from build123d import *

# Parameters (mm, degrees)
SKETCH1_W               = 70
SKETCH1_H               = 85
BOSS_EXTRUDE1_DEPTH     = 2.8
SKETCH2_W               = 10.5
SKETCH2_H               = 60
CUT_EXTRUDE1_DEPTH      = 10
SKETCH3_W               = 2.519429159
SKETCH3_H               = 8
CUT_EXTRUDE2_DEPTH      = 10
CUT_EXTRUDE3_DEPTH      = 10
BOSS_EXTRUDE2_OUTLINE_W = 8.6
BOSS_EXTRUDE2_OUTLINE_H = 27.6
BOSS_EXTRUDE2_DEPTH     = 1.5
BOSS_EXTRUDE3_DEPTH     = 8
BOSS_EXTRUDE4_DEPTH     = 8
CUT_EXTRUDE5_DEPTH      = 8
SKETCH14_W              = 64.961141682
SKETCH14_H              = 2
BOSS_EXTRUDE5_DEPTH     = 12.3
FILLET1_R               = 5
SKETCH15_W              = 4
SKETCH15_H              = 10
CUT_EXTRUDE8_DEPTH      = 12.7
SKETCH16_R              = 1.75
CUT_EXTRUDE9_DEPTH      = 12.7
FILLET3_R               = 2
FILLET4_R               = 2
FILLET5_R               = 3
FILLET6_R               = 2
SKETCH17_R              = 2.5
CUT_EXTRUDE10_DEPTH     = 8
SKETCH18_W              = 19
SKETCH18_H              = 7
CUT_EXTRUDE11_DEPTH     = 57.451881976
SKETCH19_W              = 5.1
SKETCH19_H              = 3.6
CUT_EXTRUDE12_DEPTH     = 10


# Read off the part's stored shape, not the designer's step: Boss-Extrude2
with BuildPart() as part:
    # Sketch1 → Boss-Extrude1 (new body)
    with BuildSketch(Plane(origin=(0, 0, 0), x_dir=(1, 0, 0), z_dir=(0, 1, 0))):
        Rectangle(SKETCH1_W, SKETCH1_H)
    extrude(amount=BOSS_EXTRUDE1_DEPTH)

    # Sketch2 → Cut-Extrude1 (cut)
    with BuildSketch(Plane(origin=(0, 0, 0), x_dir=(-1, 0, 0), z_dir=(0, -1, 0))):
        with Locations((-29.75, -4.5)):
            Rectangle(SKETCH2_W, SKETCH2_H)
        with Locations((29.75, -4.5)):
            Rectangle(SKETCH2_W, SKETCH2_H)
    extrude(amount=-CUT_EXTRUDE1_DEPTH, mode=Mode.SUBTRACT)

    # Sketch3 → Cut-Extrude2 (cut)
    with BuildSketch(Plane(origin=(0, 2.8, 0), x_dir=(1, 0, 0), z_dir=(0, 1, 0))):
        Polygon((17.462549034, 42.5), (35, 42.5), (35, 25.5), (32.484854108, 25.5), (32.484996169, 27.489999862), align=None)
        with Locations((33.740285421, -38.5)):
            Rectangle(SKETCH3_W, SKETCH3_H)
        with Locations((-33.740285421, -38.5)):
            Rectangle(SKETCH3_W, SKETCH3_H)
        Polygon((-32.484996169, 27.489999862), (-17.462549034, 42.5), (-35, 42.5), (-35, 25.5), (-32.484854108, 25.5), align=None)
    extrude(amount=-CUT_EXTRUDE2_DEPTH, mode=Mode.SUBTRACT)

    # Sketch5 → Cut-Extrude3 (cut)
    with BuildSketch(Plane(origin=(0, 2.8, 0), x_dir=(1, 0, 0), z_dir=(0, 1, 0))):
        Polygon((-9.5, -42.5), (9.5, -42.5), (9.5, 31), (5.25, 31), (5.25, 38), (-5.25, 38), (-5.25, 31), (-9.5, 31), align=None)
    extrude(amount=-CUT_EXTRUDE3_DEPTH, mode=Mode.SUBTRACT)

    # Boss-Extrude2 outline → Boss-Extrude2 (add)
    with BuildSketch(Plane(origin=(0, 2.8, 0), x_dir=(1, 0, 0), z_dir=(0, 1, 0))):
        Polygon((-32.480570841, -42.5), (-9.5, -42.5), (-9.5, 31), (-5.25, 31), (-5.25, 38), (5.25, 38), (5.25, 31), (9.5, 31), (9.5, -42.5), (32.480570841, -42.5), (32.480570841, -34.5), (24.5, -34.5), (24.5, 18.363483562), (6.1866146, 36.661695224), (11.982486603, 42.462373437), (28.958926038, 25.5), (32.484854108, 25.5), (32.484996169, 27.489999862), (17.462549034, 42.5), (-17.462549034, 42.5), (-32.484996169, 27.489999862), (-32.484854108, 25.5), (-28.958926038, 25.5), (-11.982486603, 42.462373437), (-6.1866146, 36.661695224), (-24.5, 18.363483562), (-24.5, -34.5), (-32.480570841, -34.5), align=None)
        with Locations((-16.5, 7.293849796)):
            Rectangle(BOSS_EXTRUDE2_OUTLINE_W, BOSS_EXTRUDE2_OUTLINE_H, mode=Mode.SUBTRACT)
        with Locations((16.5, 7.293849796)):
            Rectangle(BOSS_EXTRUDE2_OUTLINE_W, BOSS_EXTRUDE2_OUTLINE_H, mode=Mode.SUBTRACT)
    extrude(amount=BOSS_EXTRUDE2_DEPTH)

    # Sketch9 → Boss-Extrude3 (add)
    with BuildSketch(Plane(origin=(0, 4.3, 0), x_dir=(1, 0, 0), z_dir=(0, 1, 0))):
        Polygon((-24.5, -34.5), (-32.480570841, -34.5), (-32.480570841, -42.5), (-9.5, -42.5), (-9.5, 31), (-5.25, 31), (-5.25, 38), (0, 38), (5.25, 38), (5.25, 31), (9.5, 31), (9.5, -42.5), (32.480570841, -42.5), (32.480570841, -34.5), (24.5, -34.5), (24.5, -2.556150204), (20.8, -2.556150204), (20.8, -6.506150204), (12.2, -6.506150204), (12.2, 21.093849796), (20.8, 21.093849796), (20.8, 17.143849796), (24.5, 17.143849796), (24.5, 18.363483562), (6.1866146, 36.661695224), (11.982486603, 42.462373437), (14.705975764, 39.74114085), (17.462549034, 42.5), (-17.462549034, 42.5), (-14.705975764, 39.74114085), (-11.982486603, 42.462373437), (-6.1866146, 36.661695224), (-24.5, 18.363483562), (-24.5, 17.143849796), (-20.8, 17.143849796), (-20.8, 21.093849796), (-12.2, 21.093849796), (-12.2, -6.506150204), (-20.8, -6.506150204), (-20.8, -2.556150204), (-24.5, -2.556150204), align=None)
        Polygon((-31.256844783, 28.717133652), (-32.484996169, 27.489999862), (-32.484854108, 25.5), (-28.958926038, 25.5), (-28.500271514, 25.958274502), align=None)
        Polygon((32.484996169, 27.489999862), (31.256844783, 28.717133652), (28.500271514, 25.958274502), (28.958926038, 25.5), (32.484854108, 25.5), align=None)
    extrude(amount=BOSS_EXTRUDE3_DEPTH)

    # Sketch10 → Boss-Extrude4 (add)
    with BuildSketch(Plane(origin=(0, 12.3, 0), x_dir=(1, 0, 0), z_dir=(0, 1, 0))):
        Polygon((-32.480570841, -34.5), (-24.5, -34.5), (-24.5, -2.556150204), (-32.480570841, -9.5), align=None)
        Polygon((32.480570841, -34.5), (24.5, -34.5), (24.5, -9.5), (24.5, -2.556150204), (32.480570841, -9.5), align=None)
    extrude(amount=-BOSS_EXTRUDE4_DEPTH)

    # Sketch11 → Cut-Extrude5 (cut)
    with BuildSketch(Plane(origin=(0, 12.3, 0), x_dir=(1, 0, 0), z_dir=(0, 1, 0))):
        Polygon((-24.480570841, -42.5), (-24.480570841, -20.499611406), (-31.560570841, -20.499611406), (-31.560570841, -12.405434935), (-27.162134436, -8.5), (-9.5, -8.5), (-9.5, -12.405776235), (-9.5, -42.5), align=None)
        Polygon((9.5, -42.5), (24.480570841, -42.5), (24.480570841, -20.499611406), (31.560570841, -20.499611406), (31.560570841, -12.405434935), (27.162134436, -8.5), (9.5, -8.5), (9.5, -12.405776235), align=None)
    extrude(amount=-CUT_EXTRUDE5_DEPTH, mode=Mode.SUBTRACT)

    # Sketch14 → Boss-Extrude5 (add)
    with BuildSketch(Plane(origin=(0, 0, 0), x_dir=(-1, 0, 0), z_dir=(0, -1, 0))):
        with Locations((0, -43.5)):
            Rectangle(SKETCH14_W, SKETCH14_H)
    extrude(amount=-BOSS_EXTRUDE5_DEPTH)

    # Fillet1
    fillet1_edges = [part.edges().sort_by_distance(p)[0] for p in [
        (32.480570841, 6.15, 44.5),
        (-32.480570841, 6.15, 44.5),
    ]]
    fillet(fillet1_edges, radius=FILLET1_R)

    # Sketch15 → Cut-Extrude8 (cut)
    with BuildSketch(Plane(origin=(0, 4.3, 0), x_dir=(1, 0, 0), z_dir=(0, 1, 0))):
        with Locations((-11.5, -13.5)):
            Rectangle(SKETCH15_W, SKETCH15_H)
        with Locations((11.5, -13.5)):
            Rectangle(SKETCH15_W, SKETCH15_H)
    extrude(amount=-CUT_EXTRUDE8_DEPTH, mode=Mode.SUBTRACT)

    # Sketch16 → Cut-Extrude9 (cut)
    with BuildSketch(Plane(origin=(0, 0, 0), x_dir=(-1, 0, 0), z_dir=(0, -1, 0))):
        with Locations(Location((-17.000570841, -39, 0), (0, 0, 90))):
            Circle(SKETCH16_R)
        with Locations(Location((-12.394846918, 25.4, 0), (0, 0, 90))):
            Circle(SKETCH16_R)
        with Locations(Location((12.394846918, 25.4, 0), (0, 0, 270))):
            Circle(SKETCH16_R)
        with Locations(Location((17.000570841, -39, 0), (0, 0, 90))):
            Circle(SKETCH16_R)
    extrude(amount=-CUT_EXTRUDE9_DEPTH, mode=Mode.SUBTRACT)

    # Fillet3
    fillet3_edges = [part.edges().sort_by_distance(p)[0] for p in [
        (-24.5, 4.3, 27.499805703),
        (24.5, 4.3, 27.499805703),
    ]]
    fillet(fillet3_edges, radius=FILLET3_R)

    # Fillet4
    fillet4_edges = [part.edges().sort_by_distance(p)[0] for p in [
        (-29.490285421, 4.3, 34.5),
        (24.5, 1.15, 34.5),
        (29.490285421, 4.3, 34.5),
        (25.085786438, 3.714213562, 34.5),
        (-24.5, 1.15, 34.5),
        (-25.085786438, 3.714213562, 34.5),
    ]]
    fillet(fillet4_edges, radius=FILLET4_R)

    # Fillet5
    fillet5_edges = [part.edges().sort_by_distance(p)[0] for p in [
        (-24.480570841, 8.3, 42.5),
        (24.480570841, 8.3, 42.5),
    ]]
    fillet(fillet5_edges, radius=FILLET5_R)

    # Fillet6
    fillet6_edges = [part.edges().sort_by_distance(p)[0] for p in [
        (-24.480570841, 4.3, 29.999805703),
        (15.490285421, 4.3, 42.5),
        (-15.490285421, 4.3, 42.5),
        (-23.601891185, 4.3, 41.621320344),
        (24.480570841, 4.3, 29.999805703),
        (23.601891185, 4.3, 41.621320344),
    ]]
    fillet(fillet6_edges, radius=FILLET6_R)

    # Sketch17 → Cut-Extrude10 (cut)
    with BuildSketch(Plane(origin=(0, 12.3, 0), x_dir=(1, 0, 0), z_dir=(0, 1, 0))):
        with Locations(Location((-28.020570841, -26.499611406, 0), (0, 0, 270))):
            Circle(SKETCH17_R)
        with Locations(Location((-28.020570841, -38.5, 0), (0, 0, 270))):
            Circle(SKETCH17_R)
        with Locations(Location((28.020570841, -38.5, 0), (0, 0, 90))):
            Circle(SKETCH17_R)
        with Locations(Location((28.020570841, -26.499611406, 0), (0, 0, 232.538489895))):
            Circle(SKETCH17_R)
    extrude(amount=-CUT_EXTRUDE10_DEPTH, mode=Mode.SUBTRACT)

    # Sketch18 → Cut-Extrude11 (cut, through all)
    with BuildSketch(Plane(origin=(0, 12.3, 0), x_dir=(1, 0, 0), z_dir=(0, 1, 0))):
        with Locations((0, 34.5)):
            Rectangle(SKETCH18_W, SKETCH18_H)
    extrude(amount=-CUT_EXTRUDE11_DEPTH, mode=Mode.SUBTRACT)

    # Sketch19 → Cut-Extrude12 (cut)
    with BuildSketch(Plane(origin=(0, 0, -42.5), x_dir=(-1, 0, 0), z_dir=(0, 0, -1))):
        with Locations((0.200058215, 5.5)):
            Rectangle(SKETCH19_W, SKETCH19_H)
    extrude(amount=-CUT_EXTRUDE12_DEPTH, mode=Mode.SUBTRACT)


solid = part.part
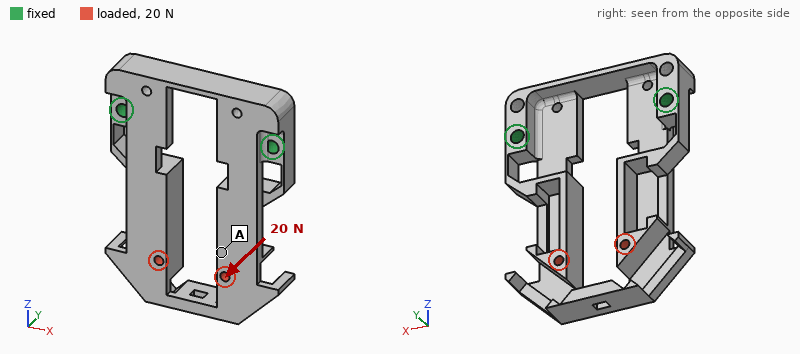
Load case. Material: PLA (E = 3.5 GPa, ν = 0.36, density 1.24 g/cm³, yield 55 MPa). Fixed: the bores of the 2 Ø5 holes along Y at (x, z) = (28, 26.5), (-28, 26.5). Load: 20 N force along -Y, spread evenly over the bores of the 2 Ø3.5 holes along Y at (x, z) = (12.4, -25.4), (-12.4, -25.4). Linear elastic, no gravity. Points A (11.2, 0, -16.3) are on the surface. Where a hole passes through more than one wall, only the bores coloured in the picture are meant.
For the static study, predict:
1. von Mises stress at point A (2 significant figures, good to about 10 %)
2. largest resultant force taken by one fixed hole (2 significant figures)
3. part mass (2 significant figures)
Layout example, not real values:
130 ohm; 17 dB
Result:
1.6 MPa; 14 N; 23 g
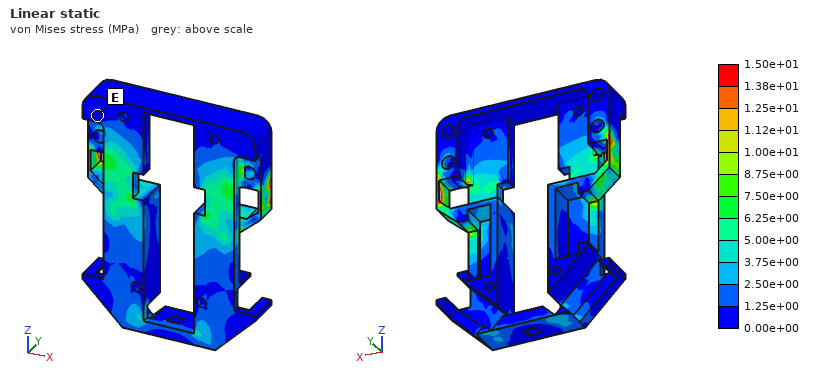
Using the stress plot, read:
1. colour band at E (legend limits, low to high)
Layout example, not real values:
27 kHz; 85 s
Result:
0.00e+00 to 1.25e+00 MPa
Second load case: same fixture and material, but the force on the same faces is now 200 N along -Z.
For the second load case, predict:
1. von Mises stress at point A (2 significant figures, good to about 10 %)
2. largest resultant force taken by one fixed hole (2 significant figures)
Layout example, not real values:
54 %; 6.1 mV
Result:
1.3 MPa; 100 N
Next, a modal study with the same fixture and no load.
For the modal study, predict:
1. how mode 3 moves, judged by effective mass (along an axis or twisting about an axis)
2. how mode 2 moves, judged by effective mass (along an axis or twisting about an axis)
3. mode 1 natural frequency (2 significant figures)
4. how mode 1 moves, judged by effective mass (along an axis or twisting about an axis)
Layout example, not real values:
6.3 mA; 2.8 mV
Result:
along X; along X; 240 Hz; along Y
